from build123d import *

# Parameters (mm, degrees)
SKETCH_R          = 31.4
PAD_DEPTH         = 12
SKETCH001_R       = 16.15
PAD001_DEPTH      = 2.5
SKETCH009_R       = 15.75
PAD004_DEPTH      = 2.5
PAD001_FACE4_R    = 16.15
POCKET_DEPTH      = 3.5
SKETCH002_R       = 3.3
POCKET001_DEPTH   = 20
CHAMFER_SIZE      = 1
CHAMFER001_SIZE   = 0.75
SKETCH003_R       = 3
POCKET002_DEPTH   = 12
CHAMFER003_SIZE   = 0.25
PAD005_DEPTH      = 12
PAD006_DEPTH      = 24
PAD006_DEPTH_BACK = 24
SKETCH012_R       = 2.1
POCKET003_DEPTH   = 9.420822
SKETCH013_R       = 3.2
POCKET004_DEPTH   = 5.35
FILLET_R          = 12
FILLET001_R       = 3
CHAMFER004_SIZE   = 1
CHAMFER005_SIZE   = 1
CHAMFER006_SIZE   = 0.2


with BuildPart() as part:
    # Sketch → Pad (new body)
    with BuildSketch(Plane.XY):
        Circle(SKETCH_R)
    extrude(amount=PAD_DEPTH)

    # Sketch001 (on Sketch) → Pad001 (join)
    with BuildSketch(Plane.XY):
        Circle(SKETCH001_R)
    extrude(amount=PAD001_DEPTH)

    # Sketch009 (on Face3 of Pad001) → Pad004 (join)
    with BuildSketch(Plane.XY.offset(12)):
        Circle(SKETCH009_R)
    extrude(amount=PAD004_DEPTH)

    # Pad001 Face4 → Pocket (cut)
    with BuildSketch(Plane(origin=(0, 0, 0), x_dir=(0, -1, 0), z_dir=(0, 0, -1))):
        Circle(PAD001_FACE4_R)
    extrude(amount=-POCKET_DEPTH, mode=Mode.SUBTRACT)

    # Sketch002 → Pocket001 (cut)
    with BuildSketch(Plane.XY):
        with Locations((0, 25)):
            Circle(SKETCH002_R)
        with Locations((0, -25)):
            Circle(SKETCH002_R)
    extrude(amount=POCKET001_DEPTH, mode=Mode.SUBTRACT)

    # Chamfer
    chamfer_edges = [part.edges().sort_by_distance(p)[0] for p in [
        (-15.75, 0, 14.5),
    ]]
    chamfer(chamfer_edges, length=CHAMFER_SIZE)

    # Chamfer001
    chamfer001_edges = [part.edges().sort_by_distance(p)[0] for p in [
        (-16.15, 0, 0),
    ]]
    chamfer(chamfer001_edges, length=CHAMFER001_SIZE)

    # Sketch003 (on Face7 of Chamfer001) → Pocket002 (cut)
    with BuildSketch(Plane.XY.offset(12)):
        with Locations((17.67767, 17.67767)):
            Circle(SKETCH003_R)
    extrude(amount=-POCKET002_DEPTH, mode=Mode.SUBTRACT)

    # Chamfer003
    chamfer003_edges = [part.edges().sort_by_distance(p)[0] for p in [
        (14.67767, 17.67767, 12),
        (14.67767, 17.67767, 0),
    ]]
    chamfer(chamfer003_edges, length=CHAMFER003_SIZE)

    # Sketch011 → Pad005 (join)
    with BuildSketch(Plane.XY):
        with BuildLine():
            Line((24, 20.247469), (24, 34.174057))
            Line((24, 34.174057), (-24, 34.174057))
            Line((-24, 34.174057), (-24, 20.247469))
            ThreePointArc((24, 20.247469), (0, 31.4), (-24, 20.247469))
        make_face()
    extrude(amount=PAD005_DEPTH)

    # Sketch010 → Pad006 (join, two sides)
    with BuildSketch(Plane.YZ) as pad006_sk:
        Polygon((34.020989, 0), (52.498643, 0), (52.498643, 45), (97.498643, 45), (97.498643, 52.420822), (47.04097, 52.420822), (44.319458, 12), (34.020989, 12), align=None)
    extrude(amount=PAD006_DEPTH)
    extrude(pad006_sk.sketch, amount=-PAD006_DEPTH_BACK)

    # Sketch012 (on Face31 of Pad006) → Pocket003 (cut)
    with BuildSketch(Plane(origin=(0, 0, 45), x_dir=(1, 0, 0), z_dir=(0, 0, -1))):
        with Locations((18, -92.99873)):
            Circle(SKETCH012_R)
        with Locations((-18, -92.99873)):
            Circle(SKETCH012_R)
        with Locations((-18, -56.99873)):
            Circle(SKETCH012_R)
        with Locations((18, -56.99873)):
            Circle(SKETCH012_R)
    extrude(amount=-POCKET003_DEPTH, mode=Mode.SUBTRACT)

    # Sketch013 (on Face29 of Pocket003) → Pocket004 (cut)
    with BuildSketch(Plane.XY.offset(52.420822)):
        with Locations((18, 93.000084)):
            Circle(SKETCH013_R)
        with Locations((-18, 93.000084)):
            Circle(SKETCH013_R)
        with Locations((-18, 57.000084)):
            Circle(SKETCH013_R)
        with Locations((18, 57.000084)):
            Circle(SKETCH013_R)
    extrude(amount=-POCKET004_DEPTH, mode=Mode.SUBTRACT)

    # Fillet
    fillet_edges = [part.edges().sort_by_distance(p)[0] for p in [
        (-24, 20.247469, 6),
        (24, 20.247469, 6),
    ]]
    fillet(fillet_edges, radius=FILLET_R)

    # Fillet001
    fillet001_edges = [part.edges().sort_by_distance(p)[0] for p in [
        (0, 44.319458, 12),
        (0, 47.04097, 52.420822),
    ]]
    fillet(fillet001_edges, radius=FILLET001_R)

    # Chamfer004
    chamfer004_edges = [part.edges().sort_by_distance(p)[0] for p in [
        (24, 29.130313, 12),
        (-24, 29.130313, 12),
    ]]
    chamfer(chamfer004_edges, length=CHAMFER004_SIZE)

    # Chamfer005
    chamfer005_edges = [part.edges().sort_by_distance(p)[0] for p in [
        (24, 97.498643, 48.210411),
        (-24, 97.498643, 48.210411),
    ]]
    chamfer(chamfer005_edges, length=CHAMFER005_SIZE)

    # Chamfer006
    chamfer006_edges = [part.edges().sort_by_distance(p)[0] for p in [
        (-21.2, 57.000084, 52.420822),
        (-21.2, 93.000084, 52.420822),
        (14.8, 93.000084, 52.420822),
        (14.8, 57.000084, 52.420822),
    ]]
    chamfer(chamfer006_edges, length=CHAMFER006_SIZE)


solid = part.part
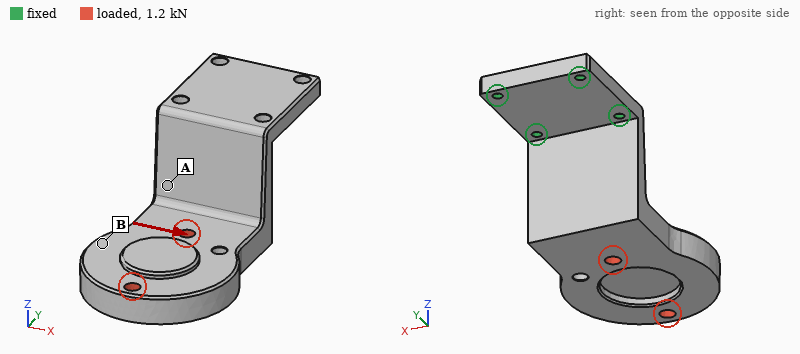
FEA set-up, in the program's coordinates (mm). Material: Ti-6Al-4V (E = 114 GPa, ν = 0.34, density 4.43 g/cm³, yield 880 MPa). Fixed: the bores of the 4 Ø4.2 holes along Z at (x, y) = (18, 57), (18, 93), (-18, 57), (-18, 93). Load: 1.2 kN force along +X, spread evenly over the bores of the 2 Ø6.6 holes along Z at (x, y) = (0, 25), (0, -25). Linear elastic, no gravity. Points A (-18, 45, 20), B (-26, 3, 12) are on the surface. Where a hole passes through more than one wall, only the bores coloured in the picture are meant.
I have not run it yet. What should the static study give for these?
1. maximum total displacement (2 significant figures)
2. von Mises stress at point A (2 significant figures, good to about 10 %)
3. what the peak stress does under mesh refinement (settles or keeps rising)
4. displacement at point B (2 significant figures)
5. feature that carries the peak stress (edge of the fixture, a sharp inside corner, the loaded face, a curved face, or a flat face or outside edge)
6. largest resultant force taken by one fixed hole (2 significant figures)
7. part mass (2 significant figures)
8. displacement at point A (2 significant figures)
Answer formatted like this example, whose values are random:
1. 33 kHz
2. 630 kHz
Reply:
1. 0.47 mm
2. 95 MPa
3. keeps rising
4. 0.31 mm
5. edge of the fixture
6. 2.2 kN
7. 340 g
8. 0.085 mm
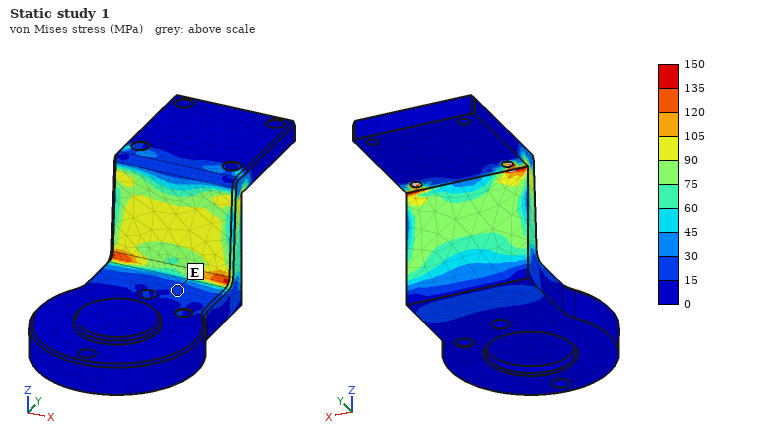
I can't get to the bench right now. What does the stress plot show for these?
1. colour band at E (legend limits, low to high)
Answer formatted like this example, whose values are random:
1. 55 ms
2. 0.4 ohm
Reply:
1. 15 to 30 MPa
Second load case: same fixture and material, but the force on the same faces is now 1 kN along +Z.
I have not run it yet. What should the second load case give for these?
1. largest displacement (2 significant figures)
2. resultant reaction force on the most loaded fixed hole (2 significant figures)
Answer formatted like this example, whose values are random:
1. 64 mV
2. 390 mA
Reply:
1. 1.5 mm
2. 2.0 kN
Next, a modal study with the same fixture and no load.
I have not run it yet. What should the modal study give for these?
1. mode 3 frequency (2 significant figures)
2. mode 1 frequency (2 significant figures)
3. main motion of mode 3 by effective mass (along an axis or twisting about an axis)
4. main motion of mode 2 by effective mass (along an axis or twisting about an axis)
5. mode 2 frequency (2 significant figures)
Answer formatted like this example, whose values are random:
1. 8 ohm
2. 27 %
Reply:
1. 1700 Hz
2. 350 Hz
3. along Y
4. along X
5. 730 Hz
